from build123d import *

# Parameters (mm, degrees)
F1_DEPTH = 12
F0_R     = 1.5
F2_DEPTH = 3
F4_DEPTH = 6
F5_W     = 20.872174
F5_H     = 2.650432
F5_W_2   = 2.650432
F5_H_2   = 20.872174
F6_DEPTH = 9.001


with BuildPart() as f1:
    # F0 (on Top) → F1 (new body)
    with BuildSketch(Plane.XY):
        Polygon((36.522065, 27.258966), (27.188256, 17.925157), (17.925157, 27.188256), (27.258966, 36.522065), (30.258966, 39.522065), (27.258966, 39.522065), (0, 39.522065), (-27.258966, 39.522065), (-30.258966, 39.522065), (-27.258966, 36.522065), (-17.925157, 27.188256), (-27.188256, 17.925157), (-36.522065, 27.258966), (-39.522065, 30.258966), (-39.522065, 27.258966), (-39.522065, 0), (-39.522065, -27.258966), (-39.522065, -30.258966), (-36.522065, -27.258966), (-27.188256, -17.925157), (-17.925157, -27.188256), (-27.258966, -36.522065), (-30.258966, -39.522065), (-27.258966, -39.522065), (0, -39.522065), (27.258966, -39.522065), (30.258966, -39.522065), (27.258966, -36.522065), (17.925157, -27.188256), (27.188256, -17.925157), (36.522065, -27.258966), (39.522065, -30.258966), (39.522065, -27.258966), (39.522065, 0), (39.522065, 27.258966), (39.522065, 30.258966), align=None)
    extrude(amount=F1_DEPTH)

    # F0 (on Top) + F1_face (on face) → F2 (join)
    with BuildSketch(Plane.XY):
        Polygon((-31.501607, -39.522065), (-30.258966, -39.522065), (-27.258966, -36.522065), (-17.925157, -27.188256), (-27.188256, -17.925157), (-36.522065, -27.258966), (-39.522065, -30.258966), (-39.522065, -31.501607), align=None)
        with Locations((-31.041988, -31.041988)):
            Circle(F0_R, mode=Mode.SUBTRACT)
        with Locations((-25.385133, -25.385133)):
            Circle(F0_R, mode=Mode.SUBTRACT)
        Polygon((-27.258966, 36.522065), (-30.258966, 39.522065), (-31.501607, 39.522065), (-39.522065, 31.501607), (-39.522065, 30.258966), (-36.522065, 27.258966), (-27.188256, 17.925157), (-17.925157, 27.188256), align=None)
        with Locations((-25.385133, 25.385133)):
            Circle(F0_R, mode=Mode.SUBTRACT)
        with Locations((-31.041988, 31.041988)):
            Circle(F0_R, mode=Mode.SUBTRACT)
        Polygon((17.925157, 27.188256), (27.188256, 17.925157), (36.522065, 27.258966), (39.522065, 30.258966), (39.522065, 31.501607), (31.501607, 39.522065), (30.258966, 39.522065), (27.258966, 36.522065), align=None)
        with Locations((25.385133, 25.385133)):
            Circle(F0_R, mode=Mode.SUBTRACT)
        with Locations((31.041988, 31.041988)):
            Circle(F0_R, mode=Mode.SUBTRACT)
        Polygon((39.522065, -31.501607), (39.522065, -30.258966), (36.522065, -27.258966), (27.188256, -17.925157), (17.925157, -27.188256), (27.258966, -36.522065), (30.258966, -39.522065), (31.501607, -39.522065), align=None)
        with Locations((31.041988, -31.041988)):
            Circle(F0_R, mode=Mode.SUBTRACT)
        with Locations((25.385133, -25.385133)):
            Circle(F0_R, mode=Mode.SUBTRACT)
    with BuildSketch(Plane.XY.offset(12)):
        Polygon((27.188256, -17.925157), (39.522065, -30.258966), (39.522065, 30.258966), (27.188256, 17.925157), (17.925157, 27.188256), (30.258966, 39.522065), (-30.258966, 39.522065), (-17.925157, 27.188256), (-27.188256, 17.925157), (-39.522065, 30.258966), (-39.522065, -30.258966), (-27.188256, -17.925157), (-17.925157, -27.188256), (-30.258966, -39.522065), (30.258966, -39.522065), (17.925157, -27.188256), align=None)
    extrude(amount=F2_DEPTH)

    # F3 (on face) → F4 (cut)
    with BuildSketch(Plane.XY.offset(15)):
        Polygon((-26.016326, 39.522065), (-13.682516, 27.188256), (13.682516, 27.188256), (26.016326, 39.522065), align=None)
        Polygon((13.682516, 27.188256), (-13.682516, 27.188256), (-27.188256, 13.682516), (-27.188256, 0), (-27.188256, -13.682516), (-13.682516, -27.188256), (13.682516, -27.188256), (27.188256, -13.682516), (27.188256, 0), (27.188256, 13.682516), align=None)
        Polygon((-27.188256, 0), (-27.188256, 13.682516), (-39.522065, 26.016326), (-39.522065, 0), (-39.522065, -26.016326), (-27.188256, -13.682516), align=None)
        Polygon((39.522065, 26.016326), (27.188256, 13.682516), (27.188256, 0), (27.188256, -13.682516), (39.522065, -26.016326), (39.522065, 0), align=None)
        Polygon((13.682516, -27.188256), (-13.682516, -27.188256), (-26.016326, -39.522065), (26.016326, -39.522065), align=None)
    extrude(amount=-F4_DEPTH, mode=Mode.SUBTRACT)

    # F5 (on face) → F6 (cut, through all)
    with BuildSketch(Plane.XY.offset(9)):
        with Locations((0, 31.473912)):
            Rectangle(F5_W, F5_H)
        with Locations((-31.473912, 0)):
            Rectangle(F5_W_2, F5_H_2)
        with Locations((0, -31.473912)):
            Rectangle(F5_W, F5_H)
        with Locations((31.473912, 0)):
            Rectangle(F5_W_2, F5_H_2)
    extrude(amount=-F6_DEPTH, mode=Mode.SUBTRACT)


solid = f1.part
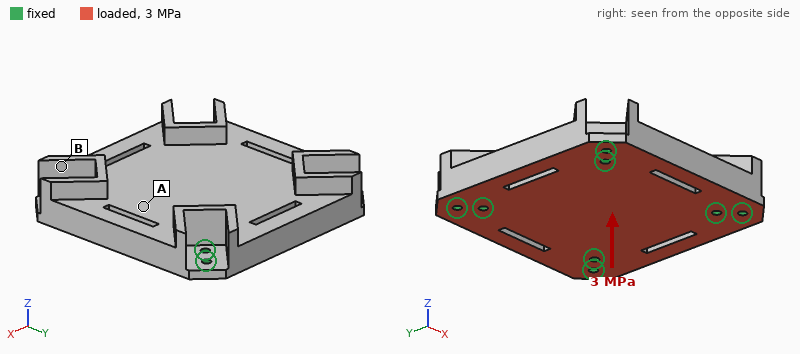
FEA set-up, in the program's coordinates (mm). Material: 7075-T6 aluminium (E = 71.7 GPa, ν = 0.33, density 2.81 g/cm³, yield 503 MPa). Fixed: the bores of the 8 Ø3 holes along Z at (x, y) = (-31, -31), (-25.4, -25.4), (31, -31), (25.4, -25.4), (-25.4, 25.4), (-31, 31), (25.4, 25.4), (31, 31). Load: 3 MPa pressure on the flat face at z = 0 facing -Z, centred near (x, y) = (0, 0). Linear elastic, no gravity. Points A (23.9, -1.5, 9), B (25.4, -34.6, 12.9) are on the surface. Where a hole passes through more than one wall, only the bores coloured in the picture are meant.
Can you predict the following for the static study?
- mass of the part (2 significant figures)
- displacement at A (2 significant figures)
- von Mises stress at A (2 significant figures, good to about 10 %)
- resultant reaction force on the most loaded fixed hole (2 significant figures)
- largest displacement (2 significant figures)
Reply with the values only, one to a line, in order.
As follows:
140 g
58 µm
47 MPa
4.0 kN
75 µm
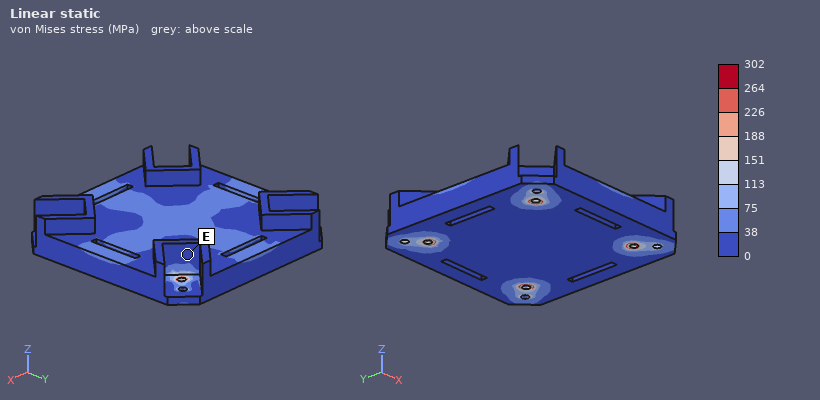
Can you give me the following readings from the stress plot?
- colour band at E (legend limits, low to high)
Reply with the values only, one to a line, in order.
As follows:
0 to 38 MPa
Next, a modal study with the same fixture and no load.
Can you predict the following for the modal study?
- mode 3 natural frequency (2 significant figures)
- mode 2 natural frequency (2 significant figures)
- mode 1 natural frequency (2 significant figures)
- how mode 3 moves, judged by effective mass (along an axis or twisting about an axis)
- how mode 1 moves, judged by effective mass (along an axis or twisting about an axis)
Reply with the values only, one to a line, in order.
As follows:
9200 Hz
8800 Hz
7300 Hz
twisting about X
along Z
